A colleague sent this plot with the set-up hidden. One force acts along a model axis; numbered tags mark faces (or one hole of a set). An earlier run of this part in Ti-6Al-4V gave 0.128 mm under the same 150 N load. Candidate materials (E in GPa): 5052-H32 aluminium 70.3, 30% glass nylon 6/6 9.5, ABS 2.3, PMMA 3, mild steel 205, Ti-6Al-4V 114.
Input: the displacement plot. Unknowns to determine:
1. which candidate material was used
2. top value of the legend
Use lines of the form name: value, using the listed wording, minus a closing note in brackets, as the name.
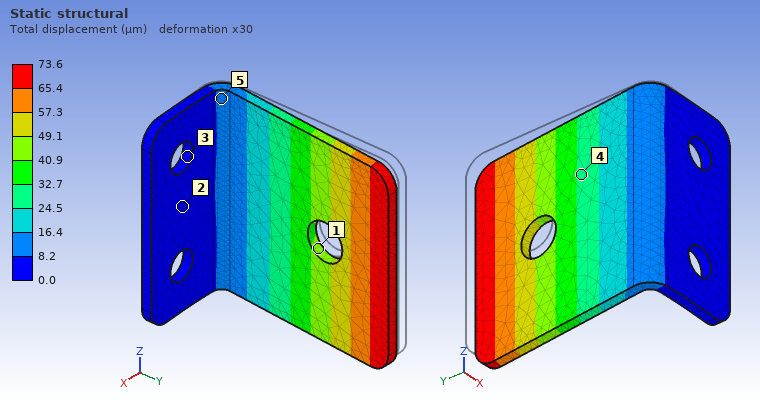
which candidate material was used: mild steel
top value of the legend: 73.6 µm
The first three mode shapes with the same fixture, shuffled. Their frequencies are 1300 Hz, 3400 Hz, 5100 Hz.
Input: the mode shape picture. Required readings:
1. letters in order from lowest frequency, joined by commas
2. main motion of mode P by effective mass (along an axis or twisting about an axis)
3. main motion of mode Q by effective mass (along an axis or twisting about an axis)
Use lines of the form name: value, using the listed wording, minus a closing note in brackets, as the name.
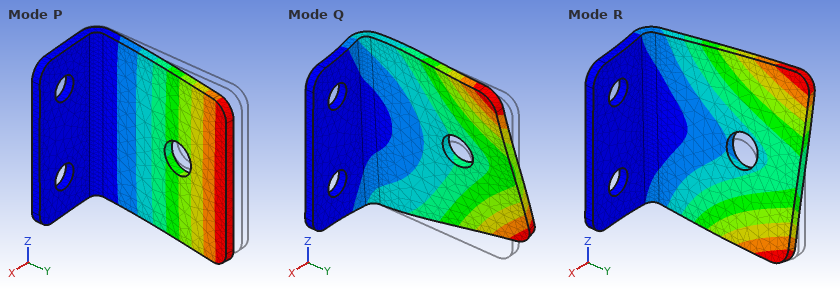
letters in order from lowest frequency, joined by commas: P, R, Q
main motion of mode P by effective mass: along X
main motion of mode Q by effective mass: along Z
